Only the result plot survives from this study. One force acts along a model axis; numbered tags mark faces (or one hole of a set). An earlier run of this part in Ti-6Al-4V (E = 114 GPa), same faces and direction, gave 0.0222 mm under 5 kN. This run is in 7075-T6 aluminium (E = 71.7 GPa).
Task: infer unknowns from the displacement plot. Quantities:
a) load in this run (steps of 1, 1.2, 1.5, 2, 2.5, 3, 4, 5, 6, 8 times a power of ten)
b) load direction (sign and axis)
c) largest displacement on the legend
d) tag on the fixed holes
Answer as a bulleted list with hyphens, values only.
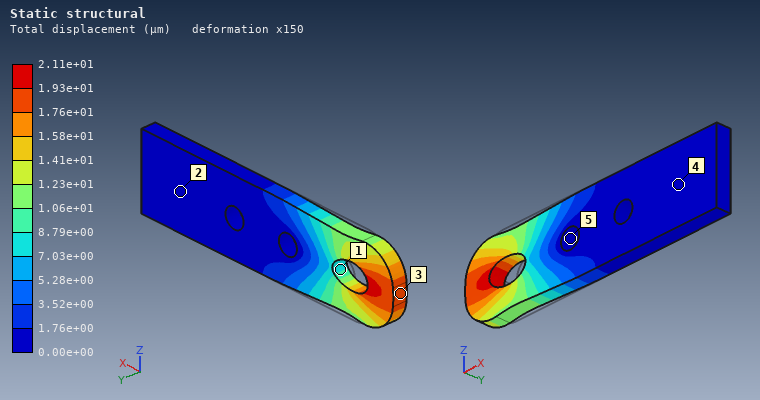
- 3 kN
- -X
- 2.11e+01 µm
- 5
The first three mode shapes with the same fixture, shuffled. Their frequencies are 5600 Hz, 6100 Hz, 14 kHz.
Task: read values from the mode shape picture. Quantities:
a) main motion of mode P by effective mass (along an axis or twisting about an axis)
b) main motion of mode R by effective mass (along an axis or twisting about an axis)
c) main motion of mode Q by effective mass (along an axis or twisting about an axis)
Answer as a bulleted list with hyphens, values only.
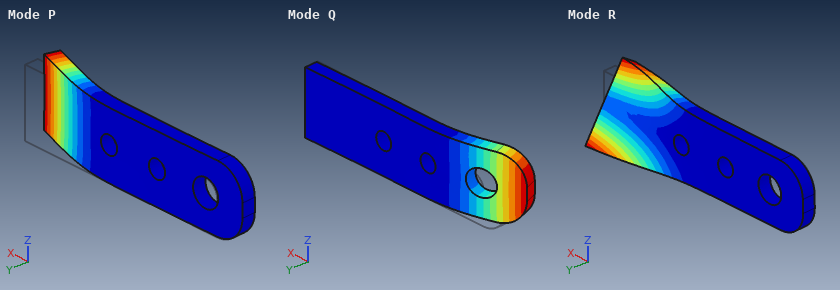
- along Y
- twisting about X
- along Y
